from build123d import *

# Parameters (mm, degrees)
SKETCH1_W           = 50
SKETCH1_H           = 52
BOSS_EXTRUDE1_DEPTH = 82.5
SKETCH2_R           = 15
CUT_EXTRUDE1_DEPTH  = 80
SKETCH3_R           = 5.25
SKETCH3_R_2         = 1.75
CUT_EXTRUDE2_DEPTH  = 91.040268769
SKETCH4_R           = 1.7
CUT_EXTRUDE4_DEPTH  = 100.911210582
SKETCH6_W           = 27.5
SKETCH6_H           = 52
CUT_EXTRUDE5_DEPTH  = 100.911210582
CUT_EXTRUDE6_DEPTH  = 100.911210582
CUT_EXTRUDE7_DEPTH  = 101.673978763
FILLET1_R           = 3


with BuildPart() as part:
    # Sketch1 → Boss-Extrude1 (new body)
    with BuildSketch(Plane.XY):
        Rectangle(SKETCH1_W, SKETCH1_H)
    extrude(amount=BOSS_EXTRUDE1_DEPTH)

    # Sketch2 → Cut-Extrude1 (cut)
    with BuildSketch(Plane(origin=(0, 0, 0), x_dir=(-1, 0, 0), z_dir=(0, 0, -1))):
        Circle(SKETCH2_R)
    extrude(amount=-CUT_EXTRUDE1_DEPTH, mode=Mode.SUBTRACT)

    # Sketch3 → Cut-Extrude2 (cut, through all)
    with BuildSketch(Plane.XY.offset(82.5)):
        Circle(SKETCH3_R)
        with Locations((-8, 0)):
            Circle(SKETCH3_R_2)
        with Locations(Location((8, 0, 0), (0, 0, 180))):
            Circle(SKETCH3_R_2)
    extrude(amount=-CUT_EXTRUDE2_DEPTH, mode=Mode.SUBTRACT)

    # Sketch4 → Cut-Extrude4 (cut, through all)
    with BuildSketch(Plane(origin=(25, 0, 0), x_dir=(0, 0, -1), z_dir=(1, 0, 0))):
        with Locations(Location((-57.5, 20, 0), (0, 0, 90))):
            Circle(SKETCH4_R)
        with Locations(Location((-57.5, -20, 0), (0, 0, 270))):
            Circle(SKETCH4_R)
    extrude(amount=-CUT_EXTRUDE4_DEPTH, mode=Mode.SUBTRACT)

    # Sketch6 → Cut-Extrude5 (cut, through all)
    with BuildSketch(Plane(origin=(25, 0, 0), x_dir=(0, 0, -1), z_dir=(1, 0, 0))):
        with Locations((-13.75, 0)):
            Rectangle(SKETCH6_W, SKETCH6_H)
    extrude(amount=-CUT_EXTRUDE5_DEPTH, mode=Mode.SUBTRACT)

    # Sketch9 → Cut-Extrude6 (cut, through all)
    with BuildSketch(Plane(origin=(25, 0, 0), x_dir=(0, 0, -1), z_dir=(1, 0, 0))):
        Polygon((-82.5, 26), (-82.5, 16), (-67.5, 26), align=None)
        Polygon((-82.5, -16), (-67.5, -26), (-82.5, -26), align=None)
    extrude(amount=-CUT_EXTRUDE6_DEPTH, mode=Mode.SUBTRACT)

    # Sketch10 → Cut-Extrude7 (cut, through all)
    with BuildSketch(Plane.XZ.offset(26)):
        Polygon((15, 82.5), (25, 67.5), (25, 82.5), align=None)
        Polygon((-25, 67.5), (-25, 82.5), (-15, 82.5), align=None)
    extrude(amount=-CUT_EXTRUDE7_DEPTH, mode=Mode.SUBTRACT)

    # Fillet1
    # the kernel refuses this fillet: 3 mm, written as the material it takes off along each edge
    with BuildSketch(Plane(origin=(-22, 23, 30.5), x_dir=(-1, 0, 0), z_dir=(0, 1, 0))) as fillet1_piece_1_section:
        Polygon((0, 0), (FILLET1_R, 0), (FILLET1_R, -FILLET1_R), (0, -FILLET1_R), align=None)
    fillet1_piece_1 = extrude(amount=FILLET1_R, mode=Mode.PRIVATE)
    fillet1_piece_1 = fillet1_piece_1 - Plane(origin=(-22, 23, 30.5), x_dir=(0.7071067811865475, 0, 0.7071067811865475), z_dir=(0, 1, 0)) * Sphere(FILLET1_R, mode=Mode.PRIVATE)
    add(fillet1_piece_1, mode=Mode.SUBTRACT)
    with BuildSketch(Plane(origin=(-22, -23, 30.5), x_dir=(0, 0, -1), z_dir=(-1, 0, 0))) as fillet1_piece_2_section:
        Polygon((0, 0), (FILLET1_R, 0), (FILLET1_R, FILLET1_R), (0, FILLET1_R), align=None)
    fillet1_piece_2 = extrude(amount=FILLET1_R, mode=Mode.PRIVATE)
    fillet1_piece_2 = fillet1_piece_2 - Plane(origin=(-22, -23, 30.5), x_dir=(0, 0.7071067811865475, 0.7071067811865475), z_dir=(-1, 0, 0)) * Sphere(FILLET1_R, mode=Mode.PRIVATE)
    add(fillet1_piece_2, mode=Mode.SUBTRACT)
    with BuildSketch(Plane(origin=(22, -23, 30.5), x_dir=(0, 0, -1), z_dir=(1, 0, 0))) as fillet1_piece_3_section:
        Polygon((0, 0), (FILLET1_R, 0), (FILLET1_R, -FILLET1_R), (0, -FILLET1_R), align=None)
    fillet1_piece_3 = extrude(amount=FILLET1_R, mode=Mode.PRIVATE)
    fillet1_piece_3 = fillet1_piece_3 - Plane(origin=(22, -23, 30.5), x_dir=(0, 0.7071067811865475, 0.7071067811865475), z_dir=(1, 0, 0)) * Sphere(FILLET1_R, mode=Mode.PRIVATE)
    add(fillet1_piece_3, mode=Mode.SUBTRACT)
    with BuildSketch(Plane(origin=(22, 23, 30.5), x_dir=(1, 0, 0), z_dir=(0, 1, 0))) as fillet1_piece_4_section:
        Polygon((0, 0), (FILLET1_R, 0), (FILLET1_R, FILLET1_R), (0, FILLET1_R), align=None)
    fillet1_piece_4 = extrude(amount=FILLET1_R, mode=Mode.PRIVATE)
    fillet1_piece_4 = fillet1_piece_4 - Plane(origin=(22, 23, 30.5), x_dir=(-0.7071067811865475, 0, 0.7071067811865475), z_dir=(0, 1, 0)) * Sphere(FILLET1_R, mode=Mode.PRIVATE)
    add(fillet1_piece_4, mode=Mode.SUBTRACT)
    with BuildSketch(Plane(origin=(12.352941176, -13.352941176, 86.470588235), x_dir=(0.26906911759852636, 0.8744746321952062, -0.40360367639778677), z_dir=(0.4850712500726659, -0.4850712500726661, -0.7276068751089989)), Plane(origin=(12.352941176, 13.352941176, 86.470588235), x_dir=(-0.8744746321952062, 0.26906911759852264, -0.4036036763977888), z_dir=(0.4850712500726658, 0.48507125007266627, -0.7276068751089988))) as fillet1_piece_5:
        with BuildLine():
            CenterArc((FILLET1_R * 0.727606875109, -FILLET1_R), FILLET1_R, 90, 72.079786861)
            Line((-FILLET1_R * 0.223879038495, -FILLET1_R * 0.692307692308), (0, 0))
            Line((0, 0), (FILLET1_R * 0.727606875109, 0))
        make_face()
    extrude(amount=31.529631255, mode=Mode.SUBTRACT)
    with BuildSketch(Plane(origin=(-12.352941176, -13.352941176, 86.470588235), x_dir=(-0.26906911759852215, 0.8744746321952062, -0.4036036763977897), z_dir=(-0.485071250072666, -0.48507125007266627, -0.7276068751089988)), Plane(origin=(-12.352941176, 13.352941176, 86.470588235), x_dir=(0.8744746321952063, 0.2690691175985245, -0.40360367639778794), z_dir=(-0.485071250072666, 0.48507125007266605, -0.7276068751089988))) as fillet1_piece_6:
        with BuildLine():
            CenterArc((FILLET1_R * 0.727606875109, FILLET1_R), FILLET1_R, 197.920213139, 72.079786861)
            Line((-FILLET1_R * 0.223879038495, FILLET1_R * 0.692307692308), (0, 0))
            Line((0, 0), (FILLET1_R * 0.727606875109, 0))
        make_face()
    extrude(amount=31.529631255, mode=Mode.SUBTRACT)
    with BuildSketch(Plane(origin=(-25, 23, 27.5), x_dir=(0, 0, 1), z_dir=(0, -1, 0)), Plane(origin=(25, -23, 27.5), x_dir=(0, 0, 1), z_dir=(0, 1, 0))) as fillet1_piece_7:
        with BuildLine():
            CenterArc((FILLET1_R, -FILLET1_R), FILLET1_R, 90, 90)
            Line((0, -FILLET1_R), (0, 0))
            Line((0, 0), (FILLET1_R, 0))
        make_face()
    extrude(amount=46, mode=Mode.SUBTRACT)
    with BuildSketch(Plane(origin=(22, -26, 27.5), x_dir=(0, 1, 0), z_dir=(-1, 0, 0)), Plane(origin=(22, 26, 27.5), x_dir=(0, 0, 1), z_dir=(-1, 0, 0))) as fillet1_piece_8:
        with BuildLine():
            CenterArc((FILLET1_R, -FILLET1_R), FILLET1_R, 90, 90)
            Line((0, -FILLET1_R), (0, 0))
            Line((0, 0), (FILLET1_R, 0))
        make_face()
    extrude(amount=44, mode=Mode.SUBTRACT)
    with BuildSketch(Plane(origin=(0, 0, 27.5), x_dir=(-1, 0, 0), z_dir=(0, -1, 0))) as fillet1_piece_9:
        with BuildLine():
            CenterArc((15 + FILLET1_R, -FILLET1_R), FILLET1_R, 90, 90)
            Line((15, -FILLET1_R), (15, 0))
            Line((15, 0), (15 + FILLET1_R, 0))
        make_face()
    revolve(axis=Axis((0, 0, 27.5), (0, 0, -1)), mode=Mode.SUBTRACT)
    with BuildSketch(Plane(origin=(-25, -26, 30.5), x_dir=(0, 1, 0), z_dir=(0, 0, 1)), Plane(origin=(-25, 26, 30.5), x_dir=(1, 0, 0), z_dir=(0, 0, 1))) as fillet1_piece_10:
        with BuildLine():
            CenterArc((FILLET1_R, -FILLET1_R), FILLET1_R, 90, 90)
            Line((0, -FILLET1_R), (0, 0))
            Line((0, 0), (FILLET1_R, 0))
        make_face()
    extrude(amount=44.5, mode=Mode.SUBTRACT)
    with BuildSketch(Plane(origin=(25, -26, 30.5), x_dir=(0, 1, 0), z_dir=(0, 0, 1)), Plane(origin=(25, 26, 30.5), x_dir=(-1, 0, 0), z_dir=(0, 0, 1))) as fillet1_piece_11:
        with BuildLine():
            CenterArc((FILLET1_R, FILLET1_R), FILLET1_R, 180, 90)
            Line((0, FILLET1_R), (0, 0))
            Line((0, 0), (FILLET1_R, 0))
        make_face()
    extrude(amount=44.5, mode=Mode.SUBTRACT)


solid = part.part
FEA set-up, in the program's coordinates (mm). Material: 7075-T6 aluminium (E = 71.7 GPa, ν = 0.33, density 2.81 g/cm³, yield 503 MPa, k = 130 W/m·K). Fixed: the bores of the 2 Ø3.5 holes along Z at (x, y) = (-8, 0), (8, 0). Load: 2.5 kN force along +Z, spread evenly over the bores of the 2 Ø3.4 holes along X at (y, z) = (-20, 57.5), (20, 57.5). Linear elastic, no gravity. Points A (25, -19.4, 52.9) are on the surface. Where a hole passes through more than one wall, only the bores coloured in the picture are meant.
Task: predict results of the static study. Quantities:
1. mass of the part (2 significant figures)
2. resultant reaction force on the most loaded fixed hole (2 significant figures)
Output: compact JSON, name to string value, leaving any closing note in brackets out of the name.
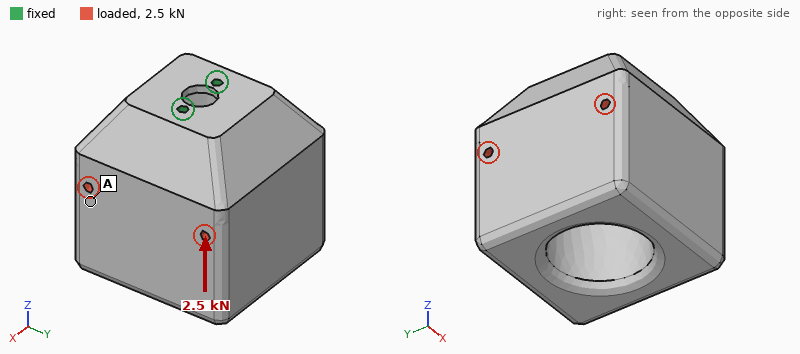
{"mass of the part": "250 g", "resultant reaction force on the most loaded fixed hole": "1.3 kN"}
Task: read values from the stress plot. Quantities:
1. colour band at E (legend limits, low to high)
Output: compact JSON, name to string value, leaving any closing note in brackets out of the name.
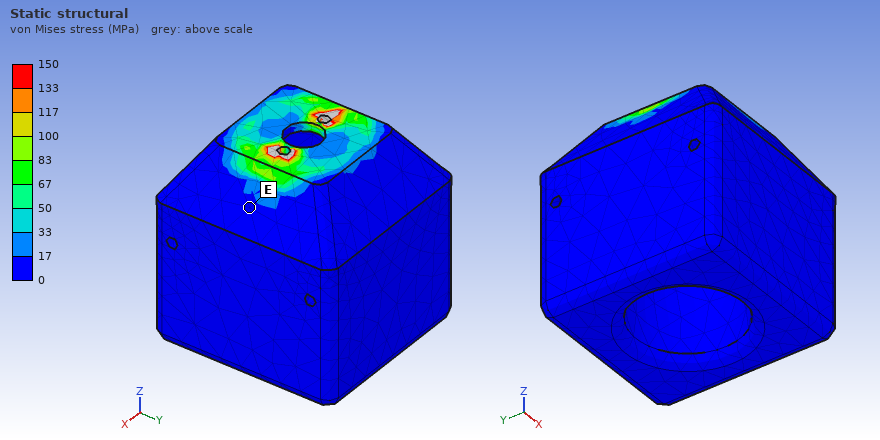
{"colour band at E": "0 to 17 MPa"}
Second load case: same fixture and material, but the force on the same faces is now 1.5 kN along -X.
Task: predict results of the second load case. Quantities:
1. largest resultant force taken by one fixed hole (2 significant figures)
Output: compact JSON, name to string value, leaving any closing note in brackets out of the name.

{"largest resultant force taken by one fixed hole": "1.7 kN"}
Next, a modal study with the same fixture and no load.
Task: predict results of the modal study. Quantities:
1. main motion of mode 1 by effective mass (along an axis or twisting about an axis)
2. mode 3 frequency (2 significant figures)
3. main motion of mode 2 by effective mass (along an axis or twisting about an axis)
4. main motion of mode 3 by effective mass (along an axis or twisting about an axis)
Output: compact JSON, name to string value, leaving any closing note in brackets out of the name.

{"main motion of mode 1 by effective mass": "along Y", "mode 3 frequency": "2600 Hz", "main motion of mode 2 by effective mass": "along X", "main motion of mode 3 by effective mass": "twisting about Z"}
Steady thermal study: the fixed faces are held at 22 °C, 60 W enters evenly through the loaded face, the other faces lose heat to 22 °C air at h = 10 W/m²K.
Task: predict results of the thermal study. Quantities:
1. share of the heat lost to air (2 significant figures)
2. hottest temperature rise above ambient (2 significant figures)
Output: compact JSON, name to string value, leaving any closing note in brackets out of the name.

{"share of the heat lost to air": "12 %", "hottest temperature rise above ambient": "43 K"}
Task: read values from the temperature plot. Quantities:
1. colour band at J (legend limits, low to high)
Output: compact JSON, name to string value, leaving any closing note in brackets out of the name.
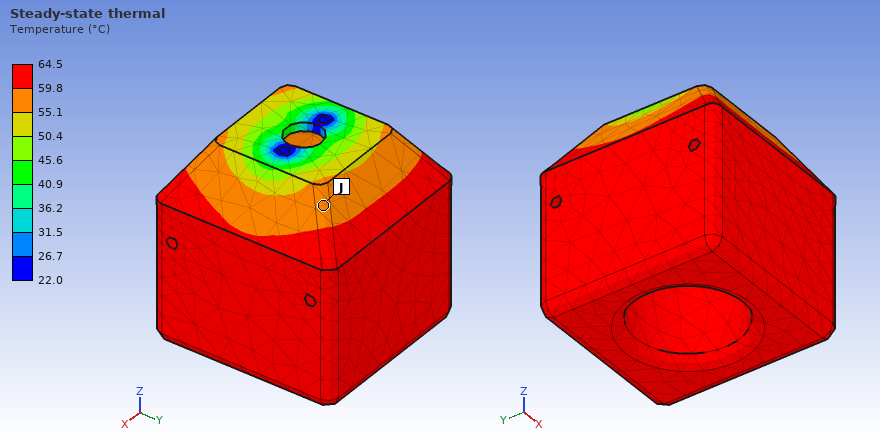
{"colour band at J": "55.1 to 59.8 °C"}
